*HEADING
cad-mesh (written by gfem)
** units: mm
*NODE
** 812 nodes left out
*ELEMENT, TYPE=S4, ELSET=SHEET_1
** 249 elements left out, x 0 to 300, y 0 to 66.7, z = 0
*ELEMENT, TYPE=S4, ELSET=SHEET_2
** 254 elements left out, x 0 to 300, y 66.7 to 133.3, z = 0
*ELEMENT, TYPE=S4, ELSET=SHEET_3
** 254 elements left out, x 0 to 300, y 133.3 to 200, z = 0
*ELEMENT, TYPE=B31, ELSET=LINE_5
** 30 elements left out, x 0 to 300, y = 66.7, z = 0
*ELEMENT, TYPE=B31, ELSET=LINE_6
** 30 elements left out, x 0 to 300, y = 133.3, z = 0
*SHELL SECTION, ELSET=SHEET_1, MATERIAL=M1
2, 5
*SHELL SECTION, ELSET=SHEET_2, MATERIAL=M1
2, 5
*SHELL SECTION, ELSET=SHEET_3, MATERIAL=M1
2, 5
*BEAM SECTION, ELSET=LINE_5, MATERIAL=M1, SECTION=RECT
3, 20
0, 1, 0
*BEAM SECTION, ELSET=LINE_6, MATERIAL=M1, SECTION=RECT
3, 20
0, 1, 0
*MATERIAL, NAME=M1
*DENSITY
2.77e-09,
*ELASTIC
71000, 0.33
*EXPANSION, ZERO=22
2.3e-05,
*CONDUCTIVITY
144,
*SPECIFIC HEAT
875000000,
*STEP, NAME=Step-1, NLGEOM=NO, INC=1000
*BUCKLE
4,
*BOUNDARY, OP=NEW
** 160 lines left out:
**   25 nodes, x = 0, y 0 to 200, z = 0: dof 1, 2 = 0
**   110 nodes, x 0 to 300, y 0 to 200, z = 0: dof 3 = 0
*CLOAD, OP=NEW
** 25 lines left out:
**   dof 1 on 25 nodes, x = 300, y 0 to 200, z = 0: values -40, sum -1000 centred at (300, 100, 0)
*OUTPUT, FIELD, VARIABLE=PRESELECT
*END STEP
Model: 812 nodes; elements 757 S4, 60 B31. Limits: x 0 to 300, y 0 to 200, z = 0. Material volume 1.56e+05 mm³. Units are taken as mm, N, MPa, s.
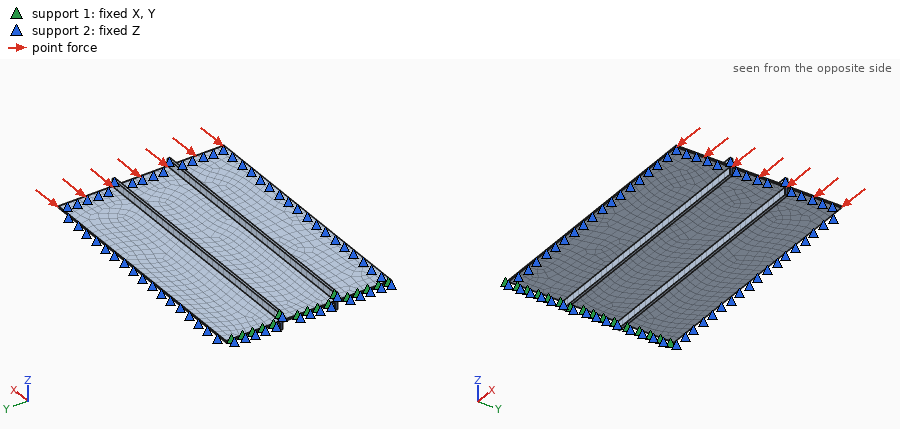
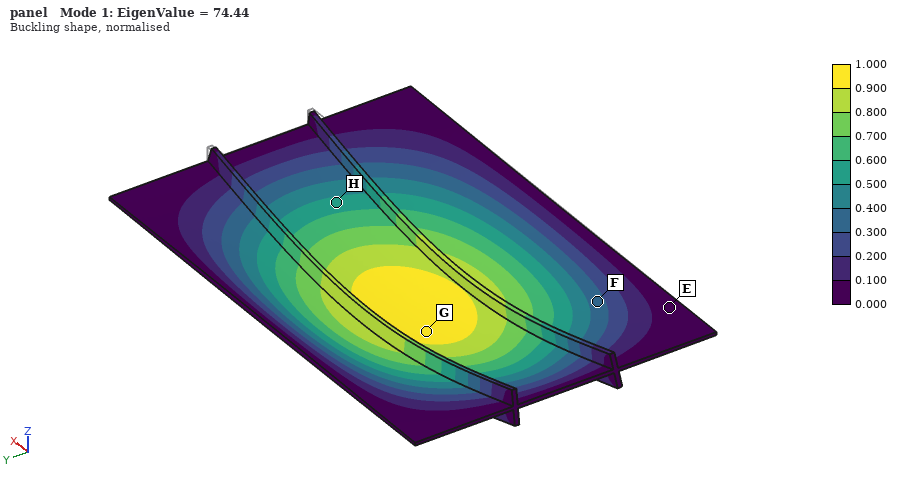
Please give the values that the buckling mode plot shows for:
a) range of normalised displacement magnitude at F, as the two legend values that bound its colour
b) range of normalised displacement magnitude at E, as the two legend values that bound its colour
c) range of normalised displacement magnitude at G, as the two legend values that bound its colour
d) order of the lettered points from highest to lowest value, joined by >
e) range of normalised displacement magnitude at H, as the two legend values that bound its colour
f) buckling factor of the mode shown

0.300 to 0.400
0.000 to 0.100
0.900 to 1.000
G > H > F > E
0.500 to 0.600
74.44
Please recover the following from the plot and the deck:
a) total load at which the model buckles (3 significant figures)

74400 N
